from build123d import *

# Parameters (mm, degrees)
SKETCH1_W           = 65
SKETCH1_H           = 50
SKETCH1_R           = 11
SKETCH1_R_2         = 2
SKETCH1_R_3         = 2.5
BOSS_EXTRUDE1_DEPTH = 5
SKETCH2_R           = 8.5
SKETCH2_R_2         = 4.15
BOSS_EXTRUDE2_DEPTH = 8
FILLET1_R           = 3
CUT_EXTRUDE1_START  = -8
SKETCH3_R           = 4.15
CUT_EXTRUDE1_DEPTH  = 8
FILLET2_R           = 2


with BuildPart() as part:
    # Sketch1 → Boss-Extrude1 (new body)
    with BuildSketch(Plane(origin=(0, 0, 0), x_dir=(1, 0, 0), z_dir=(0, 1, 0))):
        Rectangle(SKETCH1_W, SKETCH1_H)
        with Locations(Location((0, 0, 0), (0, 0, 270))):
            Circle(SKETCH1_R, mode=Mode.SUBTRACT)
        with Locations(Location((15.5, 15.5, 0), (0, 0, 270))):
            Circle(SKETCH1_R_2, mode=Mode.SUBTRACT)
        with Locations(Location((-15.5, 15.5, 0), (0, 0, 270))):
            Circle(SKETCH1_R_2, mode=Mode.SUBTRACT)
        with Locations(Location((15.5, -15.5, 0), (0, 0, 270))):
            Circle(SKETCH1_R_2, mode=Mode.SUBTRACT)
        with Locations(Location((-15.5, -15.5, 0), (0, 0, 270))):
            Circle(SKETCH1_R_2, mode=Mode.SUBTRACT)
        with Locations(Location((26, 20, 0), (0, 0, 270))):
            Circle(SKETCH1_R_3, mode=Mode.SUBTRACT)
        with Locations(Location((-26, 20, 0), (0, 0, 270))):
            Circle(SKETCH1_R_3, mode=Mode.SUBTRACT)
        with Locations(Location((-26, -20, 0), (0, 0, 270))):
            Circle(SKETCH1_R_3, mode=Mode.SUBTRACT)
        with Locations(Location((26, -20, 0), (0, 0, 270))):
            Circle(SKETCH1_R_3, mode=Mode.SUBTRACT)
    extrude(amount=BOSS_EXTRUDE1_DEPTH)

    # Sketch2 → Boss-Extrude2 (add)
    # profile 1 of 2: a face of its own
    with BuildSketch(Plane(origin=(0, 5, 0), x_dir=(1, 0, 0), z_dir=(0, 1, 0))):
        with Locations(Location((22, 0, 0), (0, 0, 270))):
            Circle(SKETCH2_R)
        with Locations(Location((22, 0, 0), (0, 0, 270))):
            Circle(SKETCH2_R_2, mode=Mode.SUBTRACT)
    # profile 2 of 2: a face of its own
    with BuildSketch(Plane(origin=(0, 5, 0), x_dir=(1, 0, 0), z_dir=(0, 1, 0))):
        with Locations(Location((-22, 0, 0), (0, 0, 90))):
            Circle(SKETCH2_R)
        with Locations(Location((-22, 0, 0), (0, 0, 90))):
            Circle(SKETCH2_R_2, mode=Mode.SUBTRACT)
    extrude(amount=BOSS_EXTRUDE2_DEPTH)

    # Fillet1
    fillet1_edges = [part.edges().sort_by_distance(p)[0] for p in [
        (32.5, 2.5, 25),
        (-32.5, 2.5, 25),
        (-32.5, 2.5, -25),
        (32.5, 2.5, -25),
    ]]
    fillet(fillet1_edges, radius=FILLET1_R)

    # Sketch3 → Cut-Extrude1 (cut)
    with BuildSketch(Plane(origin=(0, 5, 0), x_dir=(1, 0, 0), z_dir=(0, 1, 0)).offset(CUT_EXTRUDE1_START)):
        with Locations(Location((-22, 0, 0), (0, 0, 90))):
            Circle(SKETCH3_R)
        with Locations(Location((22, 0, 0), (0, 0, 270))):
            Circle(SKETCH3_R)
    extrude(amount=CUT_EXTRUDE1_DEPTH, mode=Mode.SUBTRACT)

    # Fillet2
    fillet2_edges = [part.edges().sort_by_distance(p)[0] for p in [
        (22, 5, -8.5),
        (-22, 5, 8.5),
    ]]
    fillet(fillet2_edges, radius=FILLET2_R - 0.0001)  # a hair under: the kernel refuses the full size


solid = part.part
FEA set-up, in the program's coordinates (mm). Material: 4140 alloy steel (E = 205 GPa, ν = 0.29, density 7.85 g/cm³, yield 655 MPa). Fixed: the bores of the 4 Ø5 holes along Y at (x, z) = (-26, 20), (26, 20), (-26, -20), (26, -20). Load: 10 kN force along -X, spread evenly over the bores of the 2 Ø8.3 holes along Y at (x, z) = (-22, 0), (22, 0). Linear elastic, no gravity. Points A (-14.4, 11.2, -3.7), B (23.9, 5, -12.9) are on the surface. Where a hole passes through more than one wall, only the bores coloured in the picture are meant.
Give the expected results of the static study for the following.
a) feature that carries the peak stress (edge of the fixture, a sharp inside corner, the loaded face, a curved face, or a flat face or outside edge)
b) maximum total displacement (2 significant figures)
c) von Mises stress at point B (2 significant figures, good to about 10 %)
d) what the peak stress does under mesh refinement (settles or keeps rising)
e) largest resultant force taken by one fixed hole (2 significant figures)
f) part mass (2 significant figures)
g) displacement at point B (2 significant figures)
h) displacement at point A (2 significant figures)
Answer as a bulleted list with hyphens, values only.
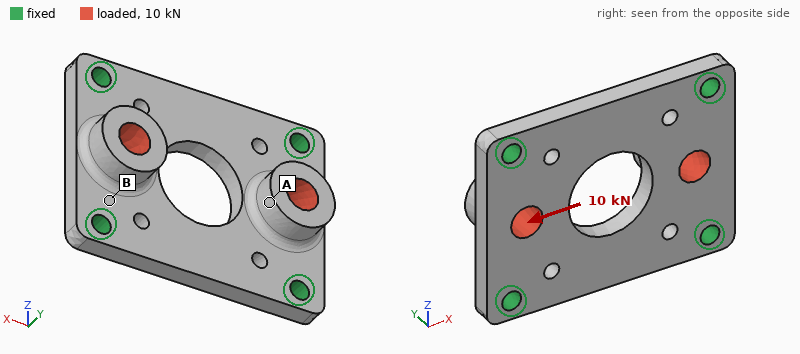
- edge of the fixture
- 20 µm
- 90 MPa
- keeps rising
- 2.6 kN
- 130 g
- 4.0 µm
- 17 µm
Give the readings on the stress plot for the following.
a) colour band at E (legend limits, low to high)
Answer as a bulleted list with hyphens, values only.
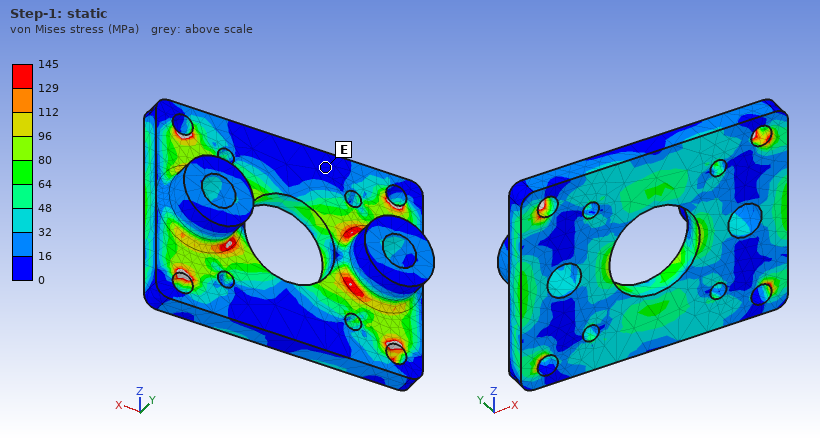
- 0 to 16 MPa
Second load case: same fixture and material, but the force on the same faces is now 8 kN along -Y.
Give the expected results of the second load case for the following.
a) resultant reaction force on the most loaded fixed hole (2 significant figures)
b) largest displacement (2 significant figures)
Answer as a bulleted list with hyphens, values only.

- 2.2 kN
- 30 µm
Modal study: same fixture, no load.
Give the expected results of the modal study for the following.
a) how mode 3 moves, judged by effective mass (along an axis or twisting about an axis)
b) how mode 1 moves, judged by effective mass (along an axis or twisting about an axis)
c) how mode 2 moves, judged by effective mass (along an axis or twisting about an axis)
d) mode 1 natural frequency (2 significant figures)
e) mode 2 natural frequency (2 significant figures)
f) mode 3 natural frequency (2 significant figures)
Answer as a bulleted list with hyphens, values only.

- twisting about Z
- along Y
- twisting about X
- 8400 Hz
- 12 kHz
- 14 kHz
